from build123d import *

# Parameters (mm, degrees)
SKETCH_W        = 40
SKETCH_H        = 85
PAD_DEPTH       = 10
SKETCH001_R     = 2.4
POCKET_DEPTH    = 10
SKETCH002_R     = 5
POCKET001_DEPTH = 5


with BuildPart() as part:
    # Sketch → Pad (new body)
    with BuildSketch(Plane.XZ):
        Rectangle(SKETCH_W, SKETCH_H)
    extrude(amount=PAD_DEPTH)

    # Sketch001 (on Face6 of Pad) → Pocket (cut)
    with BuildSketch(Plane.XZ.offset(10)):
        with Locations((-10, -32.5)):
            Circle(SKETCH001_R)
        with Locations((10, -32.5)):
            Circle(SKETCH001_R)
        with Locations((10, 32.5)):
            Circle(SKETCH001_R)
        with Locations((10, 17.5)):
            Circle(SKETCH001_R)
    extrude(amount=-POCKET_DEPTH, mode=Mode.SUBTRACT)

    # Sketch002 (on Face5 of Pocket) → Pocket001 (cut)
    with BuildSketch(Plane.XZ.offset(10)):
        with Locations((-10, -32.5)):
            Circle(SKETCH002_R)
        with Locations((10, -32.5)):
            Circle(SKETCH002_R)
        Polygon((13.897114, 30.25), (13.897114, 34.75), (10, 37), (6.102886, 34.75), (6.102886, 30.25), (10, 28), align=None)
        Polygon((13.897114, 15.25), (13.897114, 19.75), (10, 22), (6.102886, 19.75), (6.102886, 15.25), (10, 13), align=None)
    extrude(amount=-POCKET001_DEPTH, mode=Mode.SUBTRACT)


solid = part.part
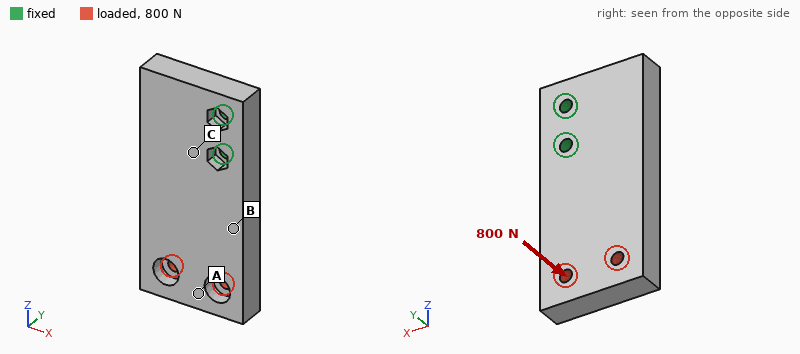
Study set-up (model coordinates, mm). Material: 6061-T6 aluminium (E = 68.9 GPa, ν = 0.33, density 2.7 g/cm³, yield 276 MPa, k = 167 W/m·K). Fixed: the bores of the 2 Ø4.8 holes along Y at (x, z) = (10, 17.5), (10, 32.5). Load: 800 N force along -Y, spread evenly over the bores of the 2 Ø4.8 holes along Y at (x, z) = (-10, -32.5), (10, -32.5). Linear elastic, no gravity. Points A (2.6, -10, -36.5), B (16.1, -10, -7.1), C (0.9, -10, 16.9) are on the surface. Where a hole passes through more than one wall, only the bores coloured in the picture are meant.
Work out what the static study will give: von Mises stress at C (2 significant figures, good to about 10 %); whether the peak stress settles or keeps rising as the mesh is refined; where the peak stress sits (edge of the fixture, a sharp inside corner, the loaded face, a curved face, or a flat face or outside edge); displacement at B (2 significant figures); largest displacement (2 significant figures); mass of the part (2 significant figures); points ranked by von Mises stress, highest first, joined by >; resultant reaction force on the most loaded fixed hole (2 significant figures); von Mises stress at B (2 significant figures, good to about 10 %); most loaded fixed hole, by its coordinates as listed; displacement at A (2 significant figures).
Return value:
64 MPa
keeps rising
edge of the fixture
0.087 mm
0.34 mm
87 g
C > B > A
2.8 kN
33 MPa
(10, 17.5)
0.28 mm
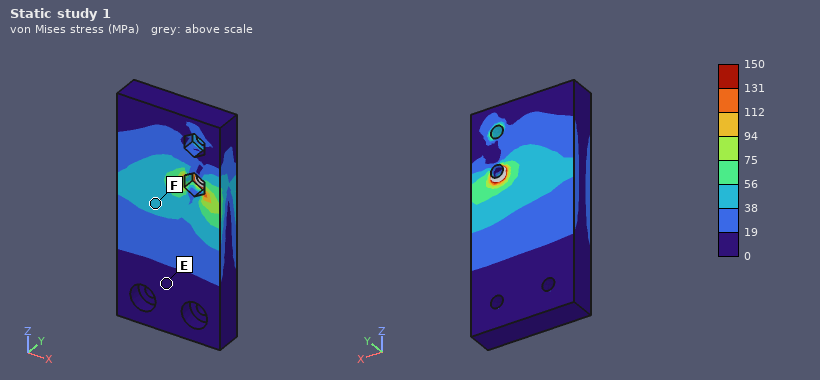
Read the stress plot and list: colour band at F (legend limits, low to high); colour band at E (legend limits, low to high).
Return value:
38 to 56 MPa
0 to 19 MPa
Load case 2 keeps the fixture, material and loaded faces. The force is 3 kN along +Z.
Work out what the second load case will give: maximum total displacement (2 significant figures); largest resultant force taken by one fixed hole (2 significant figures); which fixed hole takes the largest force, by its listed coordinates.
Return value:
79 µm
2.6 kN
(10, 17.5)
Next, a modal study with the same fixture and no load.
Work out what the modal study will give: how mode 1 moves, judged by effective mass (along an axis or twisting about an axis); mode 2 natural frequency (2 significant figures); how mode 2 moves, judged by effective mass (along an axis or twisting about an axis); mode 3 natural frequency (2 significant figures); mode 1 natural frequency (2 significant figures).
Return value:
along Y
3500 Hz
along X
3900 Hz
1700 Hz
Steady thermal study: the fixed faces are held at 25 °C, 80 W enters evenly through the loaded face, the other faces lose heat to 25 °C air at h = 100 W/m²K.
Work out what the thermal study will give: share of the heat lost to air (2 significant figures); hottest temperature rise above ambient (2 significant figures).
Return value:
33 %
65 K
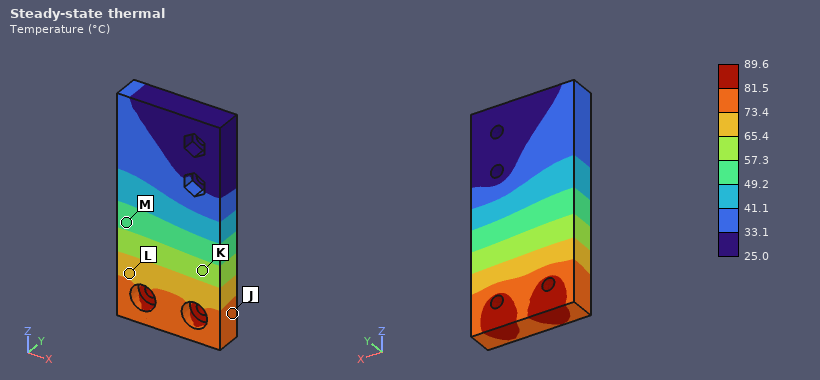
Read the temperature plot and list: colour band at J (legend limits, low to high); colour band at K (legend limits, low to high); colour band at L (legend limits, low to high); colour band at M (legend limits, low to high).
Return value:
73.4 to 81.5 °C
57.3 to 65.4 °C
65.4 to 73.4 °C
49.2 to 57.3 °C
